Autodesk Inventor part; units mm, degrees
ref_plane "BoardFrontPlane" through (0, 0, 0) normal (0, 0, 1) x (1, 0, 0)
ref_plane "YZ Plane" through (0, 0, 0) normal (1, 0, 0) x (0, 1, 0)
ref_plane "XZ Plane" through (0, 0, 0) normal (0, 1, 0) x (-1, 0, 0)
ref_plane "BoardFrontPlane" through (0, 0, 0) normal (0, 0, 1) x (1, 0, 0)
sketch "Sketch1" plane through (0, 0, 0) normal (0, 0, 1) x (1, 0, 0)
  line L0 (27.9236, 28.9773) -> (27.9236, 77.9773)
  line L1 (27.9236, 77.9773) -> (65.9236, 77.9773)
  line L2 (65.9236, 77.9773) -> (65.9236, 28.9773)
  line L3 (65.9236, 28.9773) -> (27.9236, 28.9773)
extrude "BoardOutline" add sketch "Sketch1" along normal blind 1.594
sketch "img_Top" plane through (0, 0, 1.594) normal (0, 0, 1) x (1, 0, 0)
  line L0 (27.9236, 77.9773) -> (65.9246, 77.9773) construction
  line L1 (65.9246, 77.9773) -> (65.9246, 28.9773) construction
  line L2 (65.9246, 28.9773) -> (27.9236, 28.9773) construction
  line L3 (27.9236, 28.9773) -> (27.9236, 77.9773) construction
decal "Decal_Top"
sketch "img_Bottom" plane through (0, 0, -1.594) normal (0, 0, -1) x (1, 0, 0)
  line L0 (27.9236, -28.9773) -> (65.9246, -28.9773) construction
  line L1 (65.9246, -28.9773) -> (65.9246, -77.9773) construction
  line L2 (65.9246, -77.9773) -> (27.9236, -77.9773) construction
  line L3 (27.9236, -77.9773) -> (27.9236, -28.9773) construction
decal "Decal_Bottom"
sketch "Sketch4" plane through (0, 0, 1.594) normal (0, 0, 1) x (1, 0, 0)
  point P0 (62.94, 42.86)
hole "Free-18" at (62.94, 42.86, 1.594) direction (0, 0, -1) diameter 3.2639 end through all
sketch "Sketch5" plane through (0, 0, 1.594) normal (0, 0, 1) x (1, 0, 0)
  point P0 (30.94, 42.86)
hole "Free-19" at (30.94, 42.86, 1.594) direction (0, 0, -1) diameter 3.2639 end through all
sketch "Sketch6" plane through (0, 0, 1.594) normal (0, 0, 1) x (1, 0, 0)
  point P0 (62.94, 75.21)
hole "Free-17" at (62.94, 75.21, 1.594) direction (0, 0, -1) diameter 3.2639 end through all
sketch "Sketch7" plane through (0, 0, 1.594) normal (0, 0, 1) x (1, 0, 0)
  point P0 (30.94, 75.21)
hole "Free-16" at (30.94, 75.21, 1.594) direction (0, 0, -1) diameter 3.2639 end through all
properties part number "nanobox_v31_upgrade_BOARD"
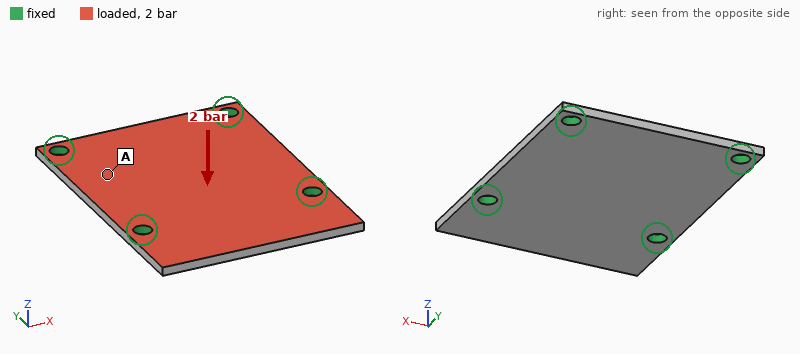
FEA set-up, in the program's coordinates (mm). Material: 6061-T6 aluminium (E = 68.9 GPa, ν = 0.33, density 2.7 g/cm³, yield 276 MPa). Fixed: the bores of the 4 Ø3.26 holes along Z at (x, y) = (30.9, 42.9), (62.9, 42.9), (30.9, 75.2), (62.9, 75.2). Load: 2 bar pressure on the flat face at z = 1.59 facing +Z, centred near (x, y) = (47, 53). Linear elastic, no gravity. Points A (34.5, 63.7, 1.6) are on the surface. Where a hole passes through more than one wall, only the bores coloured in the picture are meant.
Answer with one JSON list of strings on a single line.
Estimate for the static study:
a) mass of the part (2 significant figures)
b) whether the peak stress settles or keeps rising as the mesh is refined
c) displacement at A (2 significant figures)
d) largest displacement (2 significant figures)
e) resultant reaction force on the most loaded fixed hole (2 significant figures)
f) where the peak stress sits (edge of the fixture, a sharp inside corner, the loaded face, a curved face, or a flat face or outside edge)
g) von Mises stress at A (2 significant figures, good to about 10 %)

["7.9 g", "keeps rising", "27 µm", "65 µm", "120 N", "edge of the fixture", "17 MPa"]
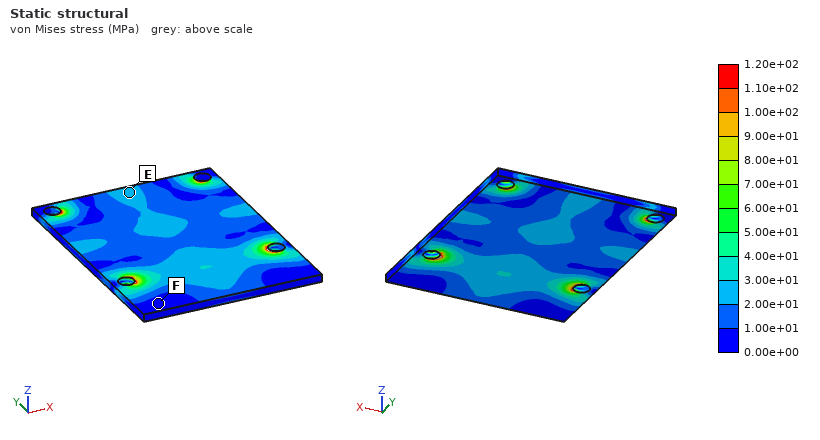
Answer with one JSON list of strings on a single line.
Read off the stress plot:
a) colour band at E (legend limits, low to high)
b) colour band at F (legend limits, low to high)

["2.00e+01 to 3.00e+01 MPa", "0.00e+00 to 1.00e+01 MPa"]
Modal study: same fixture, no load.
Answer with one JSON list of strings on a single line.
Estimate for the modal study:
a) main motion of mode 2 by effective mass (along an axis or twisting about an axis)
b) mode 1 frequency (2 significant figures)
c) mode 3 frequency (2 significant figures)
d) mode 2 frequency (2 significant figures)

["along Z", "5200 Hz", "9400 Hz", "6000 Hz"]
